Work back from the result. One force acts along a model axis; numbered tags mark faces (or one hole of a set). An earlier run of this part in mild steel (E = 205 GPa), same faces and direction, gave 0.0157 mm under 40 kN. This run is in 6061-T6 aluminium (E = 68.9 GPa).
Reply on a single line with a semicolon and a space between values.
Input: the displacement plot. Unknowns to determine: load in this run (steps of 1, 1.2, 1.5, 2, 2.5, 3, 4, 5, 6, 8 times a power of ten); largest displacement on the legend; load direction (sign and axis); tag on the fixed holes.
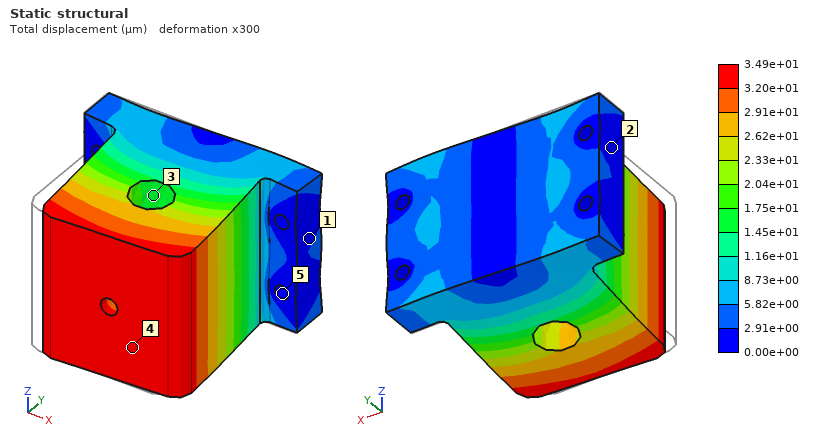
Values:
30 kN; 3.49e+01 µm; +X; 5
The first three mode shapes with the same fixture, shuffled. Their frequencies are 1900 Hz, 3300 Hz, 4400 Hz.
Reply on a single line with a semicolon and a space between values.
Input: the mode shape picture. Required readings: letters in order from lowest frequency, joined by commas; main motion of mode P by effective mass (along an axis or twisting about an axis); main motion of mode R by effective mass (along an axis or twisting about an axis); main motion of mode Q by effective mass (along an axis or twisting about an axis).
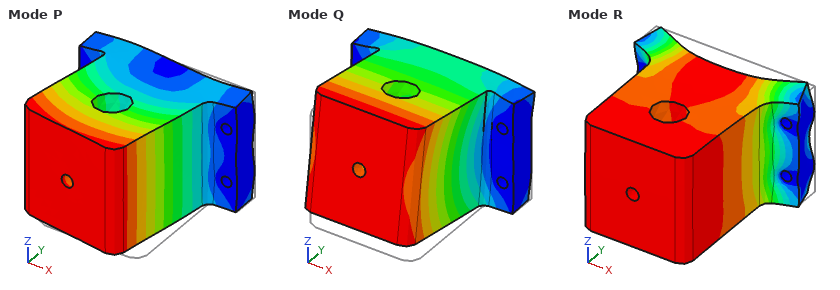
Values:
Q, P, R; along X; along Y; along Z
